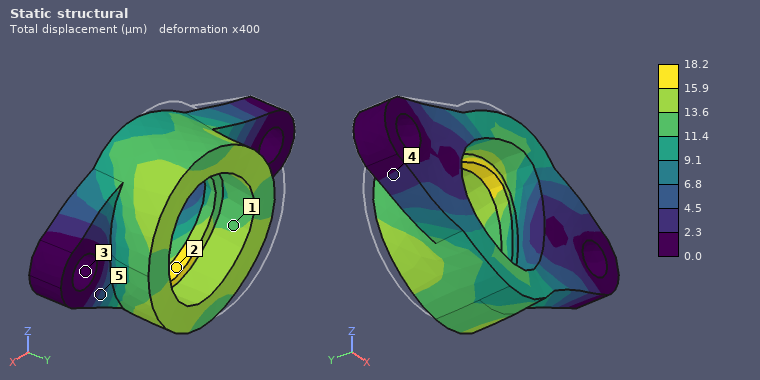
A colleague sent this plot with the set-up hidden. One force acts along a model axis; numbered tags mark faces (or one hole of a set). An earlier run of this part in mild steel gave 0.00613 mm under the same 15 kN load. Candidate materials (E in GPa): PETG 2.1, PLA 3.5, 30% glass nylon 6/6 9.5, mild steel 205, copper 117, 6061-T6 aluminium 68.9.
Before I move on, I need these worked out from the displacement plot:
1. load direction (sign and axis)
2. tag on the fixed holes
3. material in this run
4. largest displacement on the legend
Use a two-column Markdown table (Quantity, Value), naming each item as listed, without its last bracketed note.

| Quantity | Value |
|---|---|
| load direction | +X |
| tag on the fixed holes | 3 |
| material in this run | 6061-T6 aluminium |
| largest displacement on the legend | 18.2 µm |
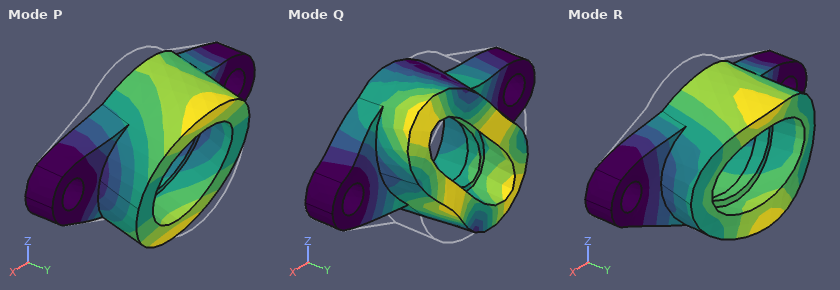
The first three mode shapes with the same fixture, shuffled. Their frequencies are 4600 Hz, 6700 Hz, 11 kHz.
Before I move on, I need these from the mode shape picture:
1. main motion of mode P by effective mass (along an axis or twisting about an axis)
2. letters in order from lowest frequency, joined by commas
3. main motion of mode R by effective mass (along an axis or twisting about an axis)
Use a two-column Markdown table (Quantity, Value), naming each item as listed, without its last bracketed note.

| Quantity | Value |
|---|---|
| main motion of mode P by effective mass | along Z |
| letters in order from lowest frequency, joined by commas | P, R, Q |
| main motion of mode R by effective mass | along Y |
